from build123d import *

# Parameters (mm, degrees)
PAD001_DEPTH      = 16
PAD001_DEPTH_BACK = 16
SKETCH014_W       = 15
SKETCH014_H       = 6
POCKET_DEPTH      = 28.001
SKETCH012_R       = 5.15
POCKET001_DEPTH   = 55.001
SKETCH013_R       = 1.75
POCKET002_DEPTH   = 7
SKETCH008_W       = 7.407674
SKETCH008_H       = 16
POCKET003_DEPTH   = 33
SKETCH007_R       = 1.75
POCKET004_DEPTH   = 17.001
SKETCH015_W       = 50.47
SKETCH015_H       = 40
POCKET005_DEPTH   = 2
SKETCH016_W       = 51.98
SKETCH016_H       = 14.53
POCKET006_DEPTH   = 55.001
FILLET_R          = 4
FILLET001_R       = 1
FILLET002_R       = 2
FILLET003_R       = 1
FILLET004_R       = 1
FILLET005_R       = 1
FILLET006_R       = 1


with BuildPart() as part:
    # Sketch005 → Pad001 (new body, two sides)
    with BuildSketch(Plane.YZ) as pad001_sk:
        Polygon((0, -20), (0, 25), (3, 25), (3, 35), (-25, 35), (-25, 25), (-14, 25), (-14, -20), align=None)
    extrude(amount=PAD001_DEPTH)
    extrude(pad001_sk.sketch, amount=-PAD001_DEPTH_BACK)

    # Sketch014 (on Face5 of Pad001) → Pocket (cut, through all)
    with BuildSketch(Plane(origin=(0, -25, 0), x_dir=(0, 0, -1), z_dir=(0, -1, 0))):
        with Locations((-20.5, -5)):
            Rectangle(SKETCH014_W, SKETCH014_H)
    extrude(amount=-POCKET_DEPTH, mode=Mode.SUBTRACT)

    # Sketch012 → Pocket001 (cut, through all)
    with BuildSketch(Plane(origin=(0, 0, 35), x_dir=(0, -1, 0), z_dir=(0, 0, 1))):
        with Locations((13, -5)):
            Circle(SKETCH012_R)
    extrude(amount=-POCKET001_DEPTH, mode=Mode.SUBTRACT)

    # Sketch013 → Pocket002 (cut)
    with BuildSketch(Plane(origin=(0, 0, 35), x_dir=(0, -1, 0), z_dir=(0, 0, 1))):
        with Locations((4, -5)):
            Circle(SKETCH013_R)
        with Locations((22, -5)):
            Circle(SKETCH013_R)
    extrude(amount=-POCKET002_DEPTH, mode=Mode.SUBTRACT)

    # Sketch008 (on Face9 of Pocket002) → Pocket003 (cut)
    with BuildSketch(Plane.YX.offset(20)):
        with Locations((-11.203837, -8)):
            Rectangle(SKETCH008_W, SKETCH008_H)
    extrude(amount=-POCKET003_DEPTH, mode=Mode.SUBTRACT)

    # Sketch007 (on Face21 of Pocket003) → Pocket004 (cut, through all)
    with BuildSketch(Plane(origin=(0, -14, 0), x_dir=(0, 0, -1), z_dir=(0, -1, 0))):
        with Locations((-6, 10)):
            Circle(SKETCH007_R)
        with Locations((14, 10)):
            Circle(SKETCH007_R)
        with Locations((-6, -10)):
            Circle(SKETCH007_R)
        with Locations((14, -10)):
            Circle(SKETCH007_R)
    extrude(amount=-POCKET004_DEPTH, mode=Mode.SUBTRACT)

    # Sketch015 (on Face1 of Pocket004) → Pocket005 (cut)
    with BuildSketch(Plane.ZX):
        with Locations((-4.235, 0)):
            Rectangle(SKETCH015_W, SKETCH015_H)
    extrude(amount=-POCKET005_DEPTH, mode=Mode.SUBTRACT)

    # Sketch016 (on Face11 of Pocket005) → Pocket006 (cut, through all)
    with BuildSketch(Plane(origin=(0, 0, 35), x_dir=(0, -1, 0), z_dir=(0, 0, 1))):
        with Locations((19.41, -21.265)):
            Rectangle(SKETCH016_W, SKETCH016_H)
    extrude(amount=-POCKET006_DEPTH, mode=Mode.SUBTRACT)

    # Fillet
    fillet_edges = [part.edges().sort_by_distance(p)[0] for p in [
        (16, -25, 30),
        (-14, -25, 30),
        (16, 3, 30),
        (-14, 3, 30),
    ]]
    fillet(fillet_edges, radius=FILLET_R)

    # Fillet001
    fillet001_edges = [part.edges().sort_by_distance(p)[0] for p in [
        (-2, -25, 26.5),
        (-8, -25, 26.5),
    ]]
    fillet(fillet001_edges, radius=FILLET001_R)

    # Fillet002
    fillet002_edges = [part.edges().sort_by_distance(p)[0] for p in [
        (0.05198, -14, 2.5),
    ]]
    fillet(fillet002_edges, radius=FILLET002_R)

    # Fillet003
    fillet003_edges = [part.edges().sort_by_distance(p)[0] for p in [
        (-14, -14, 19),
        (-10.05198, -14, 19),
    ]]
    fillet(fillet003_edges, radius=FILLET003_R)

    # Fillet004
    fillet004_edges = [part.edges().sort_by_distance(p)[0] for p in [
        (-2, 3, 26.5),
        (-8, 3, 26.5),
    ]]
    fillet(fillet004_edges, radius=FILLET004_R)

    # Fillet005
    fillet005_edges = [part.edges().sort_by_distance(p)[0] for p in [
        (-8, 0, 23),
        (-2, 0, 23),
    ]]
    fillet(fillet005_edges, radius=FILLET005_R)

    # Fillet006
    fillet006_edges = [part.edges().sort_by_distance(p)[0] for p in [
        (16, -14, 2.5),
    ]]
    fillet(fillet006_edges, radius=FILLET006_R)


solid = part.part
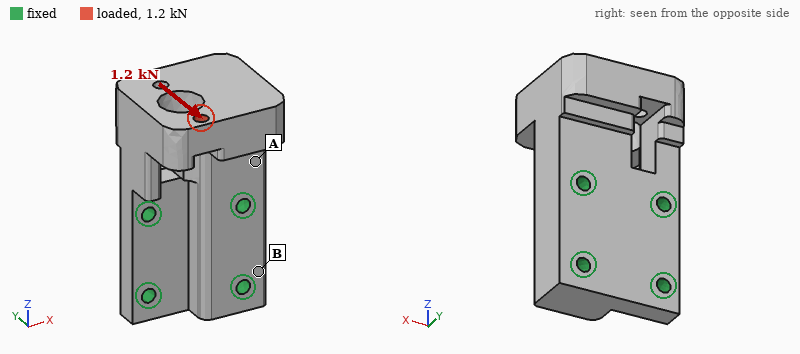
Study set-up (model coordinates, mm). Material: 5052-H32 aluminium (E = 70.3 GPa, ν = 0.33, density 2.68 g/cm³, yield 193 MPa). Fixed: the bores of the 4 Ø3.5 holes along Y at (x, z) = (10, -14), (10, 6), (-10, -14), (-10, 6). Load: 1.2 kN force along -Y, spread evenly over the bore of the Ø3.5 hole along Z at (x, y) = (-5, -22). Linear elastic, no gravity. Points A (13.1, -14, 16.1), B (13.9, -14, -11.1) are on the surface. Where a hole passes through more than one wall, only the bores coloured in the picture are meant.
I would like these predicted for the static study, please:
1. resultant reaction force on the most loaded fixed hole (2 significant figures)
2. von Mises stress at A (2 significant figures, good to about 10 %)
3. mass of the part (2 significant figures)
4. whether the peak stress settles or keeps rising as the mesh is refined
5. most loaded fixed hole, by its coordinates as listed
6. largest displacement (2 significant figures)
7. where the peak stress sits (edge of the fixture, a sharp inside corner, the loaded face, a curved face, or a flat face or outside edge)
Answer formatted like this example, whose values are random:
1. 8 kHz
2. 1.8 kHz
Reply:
1. 990 N
2. 44 MPa
3. 51 g
4. keeps rising
5. (10, 6)
6. 0.10 mm
7. edge of the fixture
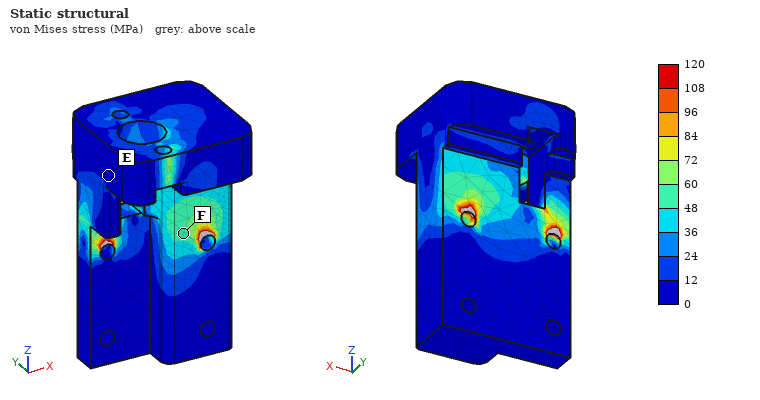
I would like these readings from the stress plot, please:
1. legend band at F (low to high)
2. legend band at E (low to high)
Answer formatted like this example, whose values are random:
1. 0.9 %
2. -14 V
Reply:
1. 48 to 60 MPa
2. 0 to 12 MPa
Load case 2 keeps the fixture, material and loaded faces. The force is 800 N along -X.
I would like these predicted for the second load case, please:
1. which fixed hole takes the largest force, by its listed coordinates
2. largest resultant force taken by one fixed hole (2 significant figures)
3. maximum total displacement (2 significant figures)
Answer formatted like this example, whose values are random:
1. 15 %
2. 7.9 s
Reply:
1. (10, 6)
2. 1.2 kN
3. 37 µm
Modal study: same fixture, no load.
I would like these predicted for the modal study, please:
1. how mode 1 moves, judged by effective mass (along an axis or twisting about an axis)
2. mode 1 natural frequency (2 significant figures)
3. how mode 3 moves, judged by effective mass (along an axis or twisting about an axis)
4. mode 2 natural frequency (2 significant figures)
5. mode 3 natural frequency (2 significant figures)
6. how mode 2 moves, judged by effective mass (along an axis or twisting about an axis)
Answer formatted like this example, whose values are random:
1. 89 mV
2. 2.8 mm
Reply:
1. along Y
2. 5200 Hz
3. along X
4. 8400 Hz
5. 11 kHz
6. along X
